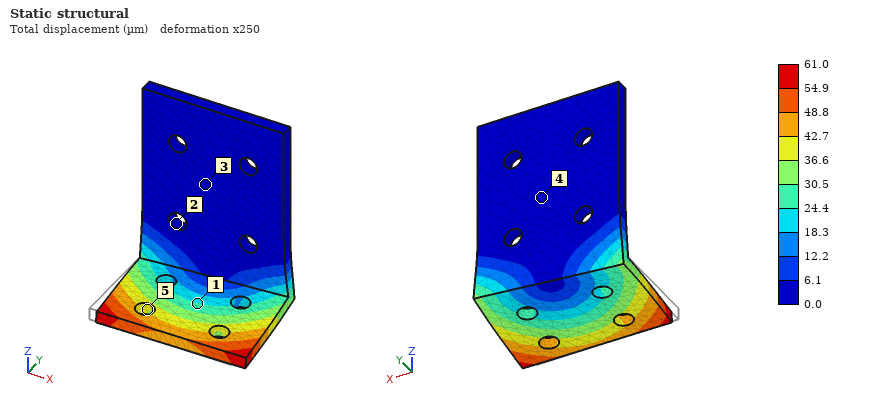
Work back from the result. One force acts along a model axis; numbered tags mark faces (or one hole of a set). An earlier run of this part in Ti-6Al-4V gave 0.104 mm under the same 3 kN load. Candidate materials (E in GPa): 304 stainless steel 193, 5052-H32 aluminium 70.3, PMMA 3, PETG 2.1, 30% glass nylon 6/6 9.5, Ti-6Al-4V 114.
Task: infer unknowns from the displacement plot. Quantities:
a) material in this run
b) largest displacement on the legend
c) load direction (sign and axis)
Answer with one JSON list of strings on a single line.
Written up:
["304 stainless steel", "61.0 µm", "+X"]
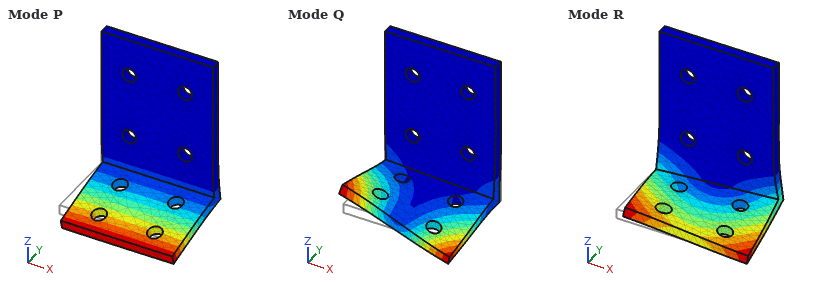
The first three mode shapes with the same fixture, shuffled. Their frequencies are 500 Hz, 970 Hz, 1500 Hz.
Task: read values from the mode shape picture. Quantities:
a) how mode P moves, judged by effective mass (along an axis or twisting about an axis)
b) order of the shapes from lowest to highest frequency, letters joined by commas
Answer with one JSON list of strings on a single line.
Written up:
["along Z", "P, R, Q"]
